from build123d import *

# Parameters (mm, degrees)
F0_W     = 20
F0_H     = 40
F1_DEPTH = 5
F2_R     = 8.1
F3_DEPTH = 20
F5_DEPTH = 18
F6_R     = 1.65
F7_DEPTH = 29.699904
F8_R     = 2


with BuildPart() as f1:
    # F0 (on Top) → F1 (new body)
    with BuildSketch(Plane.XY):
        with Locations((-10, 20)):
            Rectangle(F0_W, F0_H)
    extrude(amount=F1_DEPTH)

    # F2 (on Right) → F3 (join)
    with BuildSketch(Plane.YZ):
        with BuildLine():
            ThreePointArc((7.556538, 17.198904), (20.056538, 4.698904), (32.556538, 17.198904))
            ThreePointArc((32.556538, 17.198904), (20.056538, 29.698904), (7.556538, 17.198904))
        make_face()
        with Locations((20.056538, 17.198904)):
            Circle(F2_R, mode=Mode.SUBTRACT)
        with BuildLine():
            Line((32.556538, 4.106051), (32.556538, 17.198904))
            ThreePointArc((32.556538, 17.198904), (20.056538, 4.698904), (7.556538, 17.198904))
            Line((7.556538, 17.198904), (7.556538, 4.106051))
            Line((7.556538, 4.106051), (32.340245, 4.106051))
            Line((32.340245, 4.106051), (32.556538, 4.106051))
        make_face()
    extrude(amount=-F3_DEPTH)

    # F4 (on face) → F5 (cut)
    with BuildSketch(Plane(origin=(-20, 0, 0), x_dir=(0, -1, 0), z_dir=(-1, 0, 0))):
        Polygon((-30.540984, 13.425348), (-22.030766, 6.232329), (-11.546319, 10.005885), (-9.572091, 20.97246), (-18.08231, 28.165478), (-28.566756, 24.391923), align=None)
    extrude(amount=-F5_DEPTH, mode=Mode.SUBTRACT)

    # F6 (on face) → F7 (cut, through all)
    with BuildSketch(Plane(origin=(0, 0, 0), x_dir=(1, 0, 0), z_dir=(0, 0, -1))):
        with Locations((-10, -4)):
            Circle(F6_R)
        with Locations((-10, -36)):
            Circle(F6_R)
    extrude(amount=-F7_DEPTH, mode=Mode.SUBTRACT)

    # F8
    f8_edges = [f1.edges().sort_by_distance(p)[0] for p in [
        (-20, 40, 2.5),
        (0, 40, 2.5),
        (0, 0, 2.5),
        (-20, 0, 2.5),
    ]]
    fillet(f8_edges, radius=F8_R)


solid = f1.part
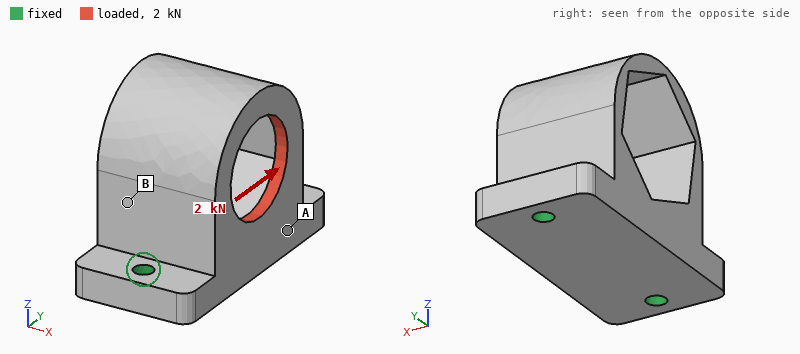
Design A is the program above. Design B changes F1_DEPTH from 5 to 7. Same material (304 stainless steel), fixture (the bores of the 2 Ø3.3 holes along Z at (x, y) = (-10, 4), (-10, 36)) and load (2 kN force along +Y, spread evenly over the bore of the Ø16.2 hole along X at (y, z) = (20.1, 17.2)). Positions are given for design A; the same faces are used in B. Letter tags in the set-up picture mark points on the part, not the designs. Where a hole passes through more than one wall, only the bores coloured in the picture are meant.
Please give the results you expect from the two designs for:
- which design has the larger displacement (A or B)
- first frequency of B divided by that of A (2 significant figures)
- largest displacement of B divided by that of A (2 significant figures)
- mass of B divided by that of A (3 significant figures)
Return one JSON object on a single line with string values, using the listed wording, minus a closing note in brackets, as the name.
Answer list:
{"which design has the larger displacement": "A", "first frequency of B divided by that of A": "1.4", "largest displacement of B divided by that of A": "0.92", "mass of B divided by that of A": "1.06"}
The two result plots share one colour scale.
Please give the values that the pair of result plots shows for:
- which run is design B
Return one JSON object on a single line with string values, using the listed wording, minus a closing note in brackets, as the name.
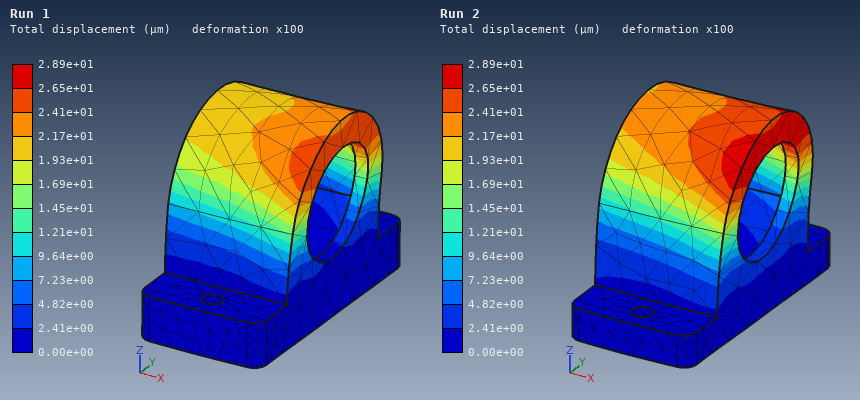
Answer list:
{"which run is design B": "Run 1"}
